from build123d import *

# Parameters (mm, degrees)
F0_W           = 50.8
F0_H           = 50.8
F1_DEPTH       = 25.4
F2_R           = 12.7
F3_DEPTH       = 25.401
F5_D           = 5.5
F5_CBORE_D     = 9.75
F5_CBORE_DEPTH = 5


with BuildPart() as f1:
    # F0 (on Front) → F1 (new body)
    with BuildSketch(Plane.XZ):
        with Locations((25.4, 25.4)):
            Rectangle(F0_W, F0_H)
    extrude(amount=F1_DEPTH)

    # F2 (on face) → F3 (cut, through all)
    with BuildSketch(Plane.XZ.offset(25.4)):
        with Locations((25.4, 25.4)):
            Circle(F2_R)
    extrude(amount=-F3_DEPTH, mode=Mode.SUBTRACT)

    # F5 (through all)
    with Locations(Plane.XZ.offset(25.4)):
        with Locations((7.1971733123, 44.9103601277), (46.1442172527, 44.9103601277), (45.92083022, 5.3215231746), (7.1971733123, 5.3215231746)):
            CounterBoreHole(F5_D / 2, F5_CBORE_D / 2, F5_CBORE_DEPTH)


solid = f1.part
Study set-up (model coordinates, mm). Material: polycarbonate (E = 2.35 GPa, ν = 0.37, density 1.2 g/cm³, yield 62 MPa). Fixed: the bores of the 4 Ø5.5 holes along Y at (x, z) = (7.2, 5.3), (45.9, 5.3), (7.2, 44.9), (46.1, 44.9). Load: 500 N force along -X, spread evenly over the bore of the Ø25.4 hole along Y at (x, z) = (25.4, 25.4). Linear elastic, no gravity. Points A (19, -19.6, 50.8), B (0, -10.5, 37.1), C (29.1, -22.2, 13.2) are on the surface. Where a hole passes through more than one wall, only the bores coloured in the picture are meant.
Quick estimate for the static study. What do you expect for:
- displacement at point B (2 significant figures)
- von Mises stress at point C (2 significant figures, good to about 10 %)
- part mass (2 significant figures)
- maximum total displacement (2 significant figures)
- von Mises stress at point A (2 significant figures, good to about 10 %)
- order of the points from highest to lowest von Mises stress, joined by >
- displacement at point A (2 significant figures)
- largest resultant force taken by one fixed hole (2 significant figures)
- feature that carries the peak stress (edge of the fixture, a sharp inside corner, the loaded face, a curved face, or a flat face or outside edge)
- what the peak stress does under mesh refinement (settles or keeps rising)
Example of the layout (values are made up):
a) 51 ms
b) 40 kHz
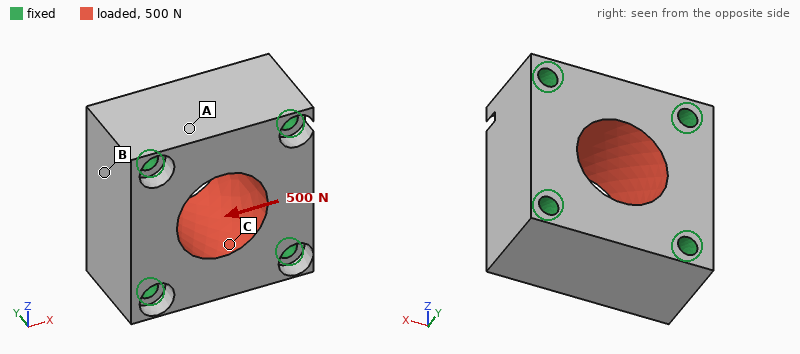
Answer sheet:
a) 2.8 µm
b) 0.50 MPa
c) 59 g
d) 6.7 µm
e) 0.23 MPa
f) C > A > B
g) 1.3 µm
h) 140 N
i) edge of the fixture
j) keeps rising
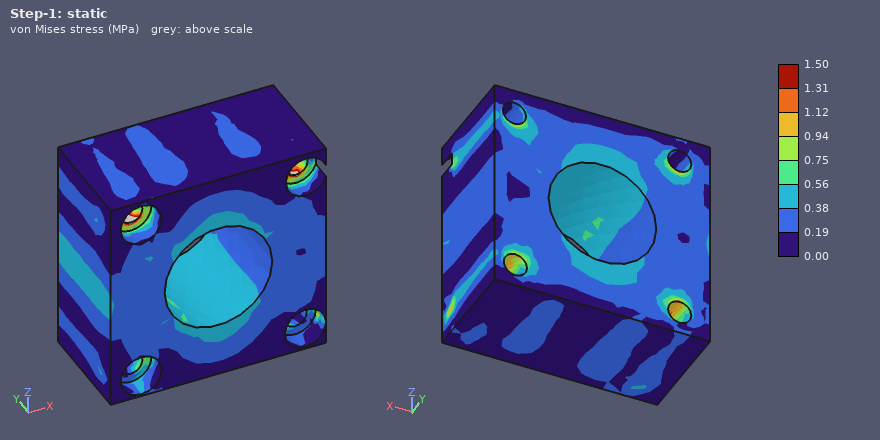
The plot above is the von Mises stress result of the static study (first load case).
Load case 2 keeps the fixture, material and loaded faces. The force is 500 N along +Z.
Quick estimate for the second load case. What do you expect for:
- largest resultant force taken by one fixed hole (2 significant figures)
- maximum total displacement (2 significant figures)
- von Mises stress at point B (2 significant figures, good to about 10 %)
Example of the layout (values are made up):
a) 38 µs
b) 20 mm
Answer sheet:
a) 140 N
b) 6.4 µm
c) 0.16 MPa
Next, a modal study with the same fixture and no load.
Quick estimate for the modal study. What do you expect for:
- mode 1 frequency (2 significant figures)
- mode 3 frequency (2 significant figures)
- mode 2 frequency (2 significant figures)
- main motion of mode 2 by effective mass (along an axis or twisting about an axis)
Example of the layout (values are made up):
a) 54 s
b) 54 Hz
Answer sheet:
a) 6700 Hz
b) 8800 Hz
c) 8100 Hz
d) along Y
